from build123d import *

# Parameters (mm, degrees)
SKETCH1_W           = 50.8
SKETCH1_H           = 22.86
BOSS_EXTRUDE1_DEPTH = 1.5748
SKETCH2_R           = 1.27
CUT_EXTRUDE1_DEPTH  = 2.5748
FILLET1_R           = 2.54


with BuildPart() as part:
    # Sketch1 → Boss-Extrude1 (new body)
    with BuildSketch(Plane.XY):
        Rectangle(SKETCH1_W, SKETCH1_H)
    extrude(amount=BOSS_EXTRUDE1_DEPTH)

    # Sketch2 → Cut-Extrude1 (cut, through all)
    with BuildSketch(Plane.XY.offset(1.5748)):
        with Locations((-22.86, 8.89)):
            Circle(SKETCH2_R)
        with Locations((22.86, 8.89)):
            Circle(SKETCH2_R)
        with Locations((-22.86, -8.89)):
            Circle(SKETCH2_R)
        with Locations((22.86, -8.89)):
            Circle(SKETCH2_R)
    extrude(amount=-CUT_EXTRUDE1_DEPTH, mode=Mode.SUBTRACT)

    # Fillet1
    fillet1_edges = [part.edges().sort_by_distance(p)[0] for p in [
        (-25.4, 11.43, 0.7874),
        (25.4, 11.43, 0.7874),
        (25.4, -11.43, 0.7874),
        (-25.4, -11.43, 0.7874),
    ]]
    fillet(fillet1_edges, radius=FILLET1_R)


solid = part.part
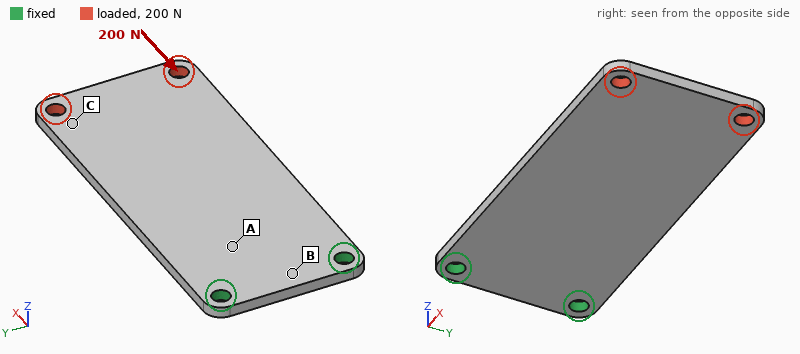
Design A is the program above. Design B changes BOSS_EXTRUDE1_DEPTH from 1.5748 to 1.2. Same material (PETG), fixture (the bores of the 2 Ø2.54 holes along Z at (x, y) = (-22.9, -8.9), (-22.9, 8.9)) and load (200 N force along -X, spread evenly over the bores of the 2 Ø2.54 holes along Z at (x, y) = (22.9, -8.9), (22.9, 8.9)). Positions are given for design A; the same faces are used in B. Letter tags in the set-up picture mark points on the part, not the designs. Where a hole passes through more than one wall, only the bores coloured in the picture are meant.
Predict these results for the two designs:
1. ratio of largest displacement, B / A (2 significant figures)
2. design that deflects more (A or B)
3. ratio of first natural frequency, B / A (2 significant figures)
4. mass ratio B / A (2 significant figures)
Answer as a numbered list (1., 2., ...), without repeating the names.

1. 1.3
2. B
3. 0.77
4. 0.76
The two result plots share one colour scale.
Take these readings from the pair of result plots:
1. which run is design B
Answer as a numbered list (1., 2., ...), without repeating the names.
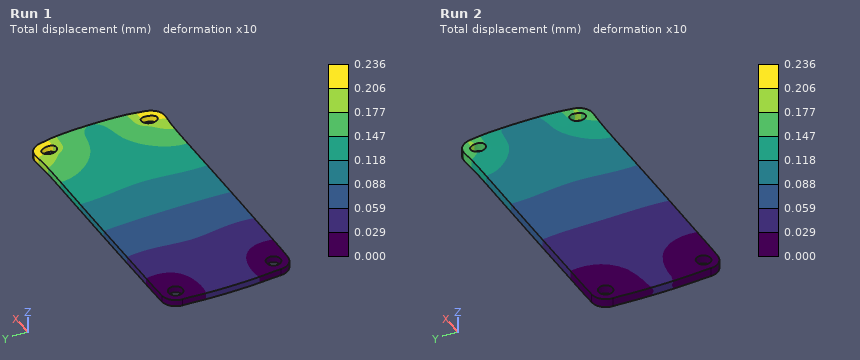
1. Run 1
